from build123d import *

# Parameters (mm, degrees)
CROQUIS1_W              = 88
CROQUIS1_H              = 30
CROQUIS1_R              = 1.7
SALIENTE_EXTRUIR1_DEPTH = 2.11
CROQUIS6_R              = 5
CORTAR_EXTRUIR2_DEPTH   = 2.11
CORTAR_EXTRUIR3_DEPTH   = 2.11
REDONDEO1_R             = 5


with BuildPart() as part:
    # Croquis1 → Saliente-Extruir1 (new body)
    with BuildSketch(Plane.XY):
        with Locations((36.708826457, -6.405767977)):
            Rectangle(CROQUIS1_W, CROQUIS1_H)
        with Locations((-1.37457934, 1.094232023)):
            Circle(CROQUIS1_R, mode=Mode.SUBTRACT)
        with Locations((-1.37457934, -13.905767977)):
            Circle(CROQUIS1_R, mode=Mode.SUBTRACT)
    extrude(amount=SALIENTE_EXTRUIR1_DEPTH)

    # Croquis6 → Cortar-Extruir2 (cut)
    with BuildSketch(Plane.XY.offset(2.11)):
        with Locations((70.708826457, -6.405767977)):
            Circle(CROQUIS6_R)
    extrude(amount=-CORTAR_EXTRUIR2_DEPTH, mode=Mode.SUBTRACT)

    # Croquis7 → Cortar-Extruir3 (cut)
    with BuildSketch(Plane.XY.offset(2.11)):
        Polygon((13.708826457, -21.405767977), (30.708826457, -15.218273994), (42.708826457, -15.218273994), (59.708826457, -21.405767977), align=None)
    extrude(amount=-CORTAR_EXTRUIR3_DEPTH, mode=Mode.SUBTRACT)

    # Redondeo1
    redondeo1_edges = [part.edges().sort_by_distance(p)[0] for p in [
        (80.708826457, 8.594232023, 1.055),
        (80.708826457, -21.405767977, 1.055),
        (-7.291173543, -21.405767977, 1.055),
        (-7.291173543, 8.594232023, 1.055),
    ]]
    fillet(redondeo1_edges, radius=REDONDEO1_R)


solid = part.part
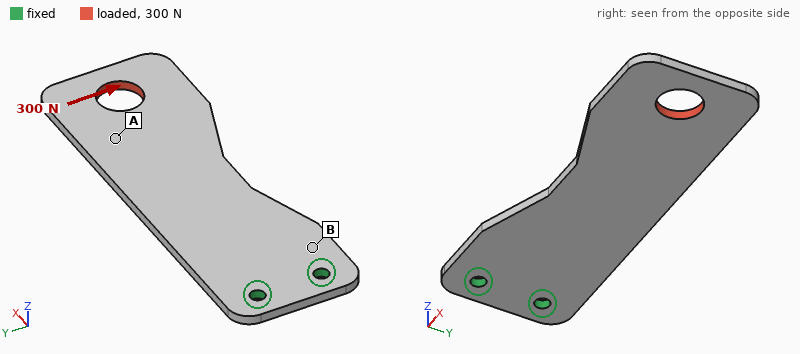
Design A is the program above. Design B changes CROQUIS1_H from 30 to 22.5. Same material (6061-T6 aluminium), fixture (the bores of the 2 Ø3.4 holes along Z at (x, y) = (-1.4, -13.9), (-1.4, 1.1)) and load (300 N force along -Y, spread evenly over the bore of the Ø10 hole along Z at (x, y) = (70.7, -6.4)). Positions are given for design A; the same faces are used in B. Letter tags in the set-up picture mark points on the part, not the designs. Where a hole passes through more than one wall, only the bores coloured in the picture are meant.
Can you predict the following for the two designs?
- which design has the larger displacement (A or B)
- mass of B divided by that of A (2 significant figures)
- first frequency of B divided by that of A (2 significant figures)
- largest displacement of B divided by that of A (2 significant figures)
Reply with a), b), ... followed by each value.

a) B
b) 0.78
c) 1.0
d) 1.6
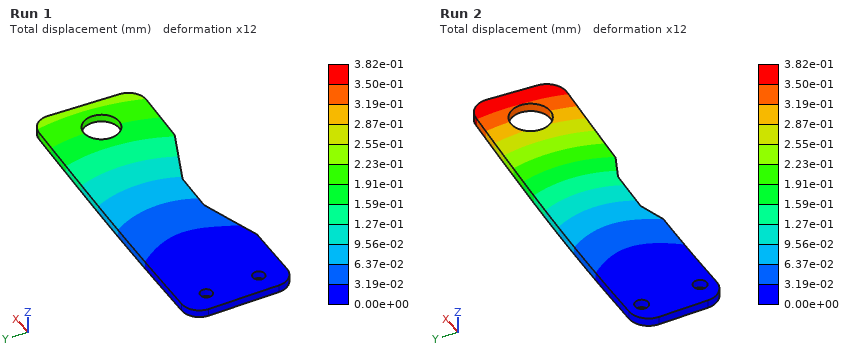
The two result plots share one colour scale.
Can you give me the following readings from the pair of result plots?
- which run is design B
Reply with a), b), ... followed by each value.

a) Run 2
